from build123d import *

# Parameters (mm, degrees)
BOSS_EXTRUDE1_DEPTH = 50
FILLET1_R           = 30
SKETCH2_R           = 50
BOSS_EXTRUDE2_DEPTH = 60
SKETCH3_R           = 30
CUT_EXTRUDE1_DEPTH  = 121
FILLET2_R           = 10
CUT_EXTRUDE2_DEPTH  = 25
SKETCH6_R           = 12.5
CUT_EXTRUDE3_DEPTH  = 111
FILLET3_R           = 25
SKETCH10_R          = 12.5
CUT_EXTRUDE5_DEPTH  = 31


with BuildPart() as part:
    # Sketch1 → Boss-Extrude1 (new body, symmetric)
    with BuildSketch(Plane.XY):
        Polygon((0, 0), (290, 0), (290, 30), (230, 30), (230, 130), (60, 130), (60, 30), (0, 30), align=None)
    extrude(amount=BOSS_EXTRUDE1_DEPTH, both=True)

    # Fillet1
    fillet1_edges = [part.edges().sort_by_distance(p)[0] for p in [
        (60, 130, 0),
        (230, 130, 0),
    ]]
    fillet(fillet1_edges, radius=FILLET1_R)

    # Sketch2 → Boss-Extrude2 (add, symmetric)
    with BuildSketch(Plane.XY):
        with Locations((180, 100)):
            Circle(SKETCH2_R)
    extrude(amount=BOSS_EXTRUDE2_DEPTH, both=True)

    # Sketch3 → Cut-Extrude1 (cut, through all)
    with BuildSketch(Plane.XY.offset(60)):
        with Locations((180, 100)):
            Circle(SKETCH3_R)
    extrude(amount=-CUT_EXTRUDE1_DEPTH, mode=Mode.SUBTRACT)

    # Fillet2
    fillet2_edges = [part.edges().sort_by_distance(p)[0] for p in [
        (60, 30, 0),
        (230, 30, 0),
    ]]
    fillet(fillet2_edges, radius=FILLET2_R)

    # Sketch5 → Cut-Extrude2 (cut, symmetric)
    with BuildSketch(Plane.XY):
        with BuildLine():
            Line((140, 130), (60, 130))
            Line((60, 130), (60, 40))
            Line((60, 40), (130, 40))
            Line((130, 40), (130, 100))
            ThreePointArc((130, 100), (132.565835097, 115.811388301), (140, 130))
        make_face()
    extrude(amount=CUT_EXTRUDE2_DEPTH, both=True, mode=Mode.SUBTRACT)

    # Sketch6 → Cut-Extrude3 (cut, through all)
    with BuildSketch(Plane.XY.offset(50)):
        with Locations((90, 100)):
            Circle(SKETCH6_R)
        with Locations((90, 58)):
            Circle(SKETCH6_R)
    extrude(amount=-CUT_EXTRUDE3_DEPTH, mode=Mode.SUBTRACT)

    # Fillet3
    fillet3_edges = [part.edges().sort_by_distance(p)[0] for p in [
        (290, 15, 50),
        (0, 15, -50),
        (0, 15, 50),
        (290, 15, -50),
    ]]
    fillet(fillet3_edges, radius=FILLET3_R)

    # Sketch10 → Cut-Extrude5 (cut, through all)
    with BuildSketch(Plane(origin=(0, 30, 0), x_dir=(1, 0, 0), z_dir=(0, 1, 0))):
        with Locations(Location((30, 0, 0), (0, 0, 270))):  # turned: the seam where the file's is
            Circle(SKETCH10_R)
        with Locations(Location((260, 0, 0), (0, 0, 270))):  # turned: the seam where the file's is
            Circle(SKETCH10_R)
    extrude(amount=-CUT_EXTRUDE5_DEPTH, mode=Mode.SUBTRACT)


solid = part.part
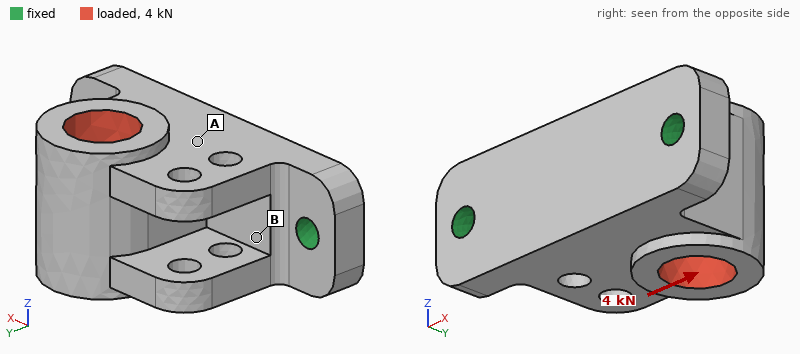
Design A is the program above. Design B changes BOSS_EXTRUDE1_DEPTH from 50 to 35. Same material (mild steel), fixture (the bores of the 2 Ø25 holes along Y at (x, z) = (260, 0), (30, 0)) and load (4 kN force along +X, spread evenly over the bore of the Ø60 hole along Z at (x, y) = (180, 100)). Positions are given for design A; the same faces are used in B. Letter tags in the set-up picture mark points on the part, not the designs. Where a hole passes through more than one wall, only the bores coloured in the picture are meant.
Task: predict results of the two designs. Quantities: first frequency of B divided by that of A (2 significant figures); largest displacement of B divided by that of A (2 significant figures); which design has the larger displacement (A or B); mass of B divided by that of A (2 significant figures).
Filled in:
0.88
1.4
B
0.74
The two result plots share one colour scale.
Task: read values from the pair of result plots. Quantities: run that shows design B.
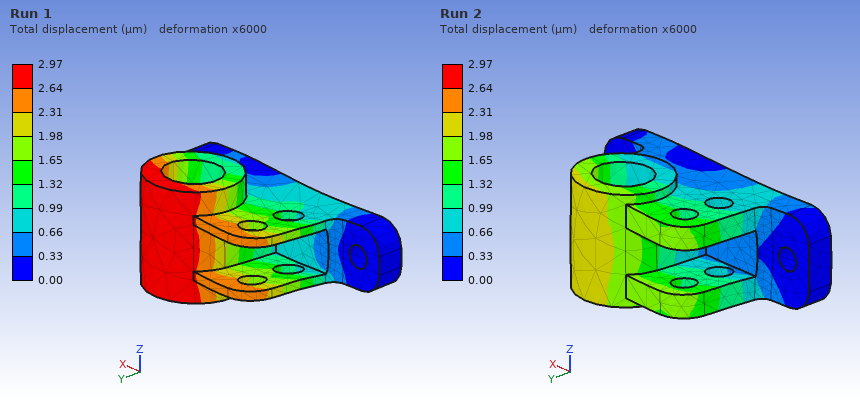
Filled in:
Run 1
